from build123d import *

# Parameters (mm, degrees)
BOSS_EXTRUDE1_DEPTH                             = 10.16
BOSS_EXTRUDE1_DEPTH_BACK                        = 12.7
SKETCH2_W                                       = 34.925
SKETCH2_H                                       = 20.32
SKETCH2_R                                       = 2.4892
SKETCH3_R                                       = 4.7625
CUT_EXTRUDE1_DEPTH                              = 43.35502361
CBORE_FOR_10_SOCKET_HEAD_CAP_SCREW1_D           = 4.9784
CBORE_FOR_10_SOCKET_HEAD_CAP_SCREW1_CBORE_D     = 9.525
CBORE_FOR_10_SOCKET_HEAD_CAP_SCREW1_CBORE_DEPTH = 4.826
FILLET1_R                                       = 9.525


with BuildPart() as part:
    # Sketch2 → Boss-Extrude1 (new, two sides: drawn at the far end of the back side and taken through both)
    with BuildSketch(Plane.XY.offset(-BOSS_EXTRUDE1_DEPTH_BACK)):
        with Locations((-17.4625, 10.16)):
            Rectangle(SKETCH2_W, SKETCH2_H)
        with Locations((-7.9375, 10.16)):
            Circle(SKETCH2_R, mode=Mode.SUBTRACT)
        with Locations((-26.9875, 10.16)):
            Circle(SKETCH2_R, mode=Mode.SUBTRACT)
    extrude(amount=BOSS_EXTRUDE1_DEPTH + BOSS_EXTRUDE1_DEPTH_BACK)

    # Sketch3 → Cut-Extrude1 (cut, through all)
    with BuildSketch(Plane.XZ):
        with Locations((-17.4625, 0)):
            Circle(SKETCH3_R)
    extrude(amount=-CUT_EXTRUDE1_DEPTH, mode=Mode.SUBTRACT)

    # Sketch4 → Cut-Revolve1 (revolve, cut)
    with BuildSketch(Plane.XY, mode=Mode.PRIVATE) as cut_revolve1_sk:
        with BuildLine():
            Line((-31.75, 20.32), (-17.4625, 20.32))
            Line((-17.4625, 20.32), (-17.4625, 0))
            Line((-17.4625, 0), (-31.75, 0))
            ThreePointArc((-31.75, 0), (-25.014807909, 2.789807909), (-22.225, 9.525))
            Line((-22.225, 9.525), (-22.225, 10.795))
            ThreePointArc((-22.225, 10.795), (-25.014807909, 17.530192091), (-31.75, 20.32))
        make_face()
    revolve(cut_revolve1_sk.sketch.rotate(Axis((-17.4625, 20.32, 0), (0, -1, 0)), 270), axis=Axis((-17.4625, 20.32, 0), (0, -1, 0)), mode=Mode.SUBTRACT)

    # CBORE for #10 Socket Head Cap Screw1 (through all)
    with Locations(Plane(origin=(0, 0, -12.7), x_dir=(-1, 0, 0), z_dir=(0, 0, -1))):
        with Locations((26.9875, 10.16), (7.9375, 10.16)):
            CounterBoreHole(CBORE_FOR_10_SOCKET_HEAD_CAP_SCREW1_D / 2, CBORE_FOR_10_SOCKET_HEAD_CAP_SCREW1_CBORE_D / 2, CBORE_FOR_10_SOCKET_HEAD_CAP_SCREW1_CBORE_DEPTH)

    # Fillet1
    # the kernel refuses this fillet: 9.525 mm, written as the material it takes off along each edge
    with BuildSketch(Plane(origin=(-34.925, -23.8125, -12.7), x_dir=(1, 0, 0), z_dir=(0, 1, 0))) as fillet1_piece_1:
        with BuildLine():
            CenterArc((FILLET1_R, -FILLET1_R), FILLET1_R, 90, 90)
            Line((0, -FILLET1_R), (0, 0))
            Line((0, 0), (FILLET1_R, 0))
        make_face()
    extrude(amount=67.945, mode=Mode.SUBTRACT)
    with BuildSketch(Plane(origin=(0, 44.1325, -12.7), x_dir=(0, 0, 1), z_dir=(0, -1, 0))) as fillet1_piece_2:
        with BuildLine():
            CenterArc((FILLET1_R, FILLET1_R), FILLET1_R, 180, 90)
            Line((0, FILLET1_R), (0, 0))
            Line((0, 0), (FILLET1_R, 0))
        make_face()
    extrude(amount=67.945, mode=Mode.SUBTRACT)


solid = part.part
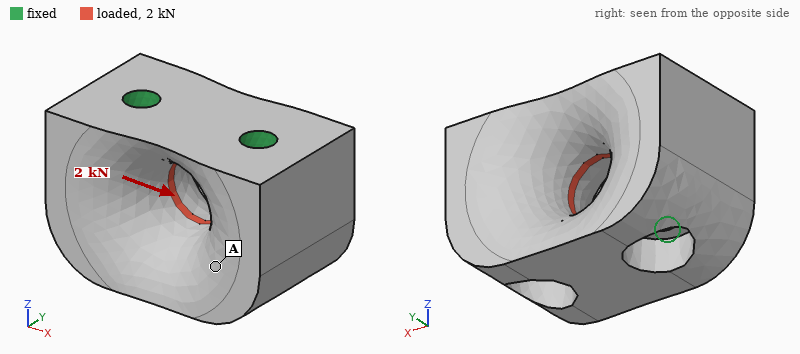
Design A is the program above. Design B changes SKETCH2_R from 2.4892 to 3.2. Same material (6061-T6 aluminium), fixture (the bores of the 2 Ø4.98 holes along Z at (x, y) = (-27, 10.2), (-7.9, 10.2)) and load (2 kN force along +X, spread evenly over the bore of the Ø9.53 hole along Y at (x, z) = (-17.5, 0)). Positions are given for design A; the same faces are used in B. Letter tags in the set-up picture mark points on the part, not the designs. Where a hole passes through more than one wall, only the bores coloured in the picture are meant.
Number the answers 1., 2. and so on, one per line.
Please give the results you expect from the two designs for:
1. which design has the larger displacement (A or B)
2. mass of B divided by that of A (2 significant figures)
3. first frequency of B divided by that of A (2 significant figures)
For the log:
1. A
2. 0.96
3. 1.1
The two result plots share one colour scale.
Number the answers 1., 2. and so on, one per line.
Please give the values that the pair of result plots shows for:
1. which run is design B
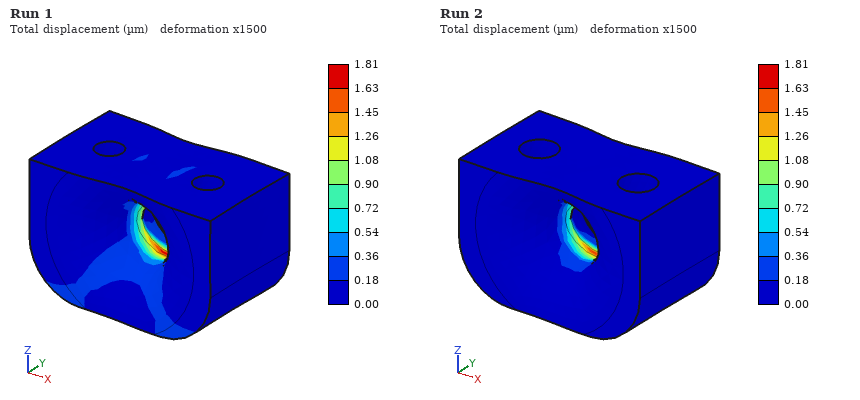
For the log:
1. Run 2
